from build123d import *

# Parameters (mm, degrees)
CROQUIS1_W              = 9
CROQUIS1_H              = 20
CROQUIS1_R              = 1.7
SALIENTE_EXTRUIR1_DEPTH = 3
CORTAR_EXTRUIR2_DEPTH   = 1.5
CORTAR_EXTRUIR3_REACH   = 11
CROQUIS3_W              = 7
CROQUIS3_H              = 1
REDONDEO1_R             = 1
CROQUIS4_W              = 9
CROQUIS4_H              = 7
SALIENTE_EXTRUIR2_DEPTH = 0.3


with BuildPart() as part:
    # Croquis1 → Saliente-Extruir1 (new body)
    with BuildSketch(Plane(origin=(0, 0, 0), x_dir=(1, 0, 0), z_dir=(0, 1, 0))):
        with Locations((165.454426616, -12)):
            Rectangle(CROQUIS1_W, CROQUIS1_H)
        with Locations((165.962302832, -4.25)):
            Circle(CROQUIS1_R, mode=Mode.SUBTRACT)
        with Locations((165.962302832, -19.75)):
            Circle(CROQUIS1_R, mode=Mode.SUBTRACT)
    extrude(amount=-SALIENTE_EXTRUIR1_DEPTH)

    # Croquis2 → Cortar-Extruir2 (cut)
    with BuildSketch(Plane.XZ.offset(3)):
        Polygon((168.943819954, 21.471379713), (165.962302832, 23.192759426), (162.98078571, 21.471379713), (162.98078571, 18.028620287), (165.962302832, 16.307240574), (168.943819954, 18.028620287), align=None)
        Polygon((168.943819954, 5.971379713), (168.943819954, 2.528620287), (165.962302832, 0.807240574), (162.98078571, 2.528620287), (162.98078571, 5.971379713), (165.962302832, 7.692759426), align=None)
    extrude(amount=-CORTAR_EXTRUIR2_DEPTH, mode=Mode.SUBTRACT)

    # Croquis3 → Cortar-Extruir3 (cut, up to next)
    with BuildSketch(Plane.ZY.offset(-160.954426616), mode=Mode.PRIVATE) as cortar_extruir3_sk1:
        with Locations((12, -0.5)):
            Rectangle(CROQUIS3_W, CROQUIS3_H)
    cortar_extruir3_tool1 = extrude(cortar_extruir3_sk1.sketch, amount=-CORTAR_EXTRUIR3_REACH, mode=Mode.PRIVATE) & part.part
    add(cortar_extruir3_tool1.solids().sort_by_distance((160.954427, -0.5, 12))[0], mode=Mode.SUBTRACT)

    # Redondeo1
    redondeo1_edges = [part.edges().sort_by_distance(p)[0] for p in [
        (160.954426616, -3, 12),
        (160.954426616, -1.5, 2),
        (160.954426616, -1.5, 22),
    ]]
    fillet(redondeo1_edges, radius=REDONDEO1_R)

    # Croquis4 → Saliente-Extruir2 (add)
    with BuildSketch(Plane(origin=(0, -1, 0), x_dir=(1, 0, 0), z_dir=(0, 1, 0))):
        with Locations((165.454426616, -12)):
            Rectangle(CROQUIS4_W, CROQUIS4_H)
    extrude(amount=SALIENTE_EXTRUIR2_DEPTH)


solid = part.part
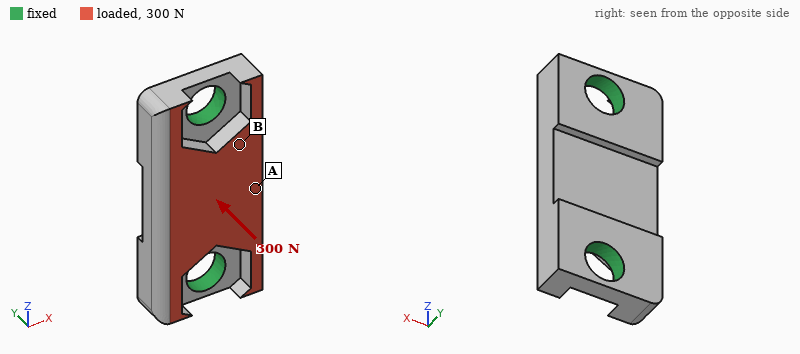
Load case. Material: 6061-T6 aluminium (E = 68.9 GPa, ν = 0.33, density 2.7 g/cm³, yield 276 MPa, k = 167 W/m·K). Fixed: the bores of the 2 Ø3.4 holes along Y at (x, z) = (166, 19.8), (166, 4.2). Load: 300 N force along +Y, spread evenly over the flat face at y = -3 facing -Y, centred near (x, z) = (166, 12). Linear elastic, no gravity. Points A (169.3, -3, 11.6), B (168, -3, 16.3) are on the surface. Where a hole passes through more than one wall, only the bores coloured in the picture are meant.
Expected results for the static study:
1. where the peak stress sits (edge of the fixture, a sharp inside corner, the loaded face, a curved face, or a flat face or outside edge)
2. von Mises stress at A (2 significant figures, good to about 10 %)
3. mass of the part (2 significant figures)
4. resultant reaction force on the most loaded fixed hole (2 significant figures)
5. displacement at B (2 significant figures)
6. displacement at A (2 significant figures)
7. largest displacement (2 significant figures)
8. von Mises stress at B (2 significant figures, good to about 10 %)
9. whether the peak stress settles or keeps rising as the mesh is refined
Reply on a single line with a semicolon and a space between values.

edge of the fixture; 28 MPa; 1.0 g; 190 N; 3.1 µm; 5.4 µm; 5.7 µm; 11 MPa; keeps rising
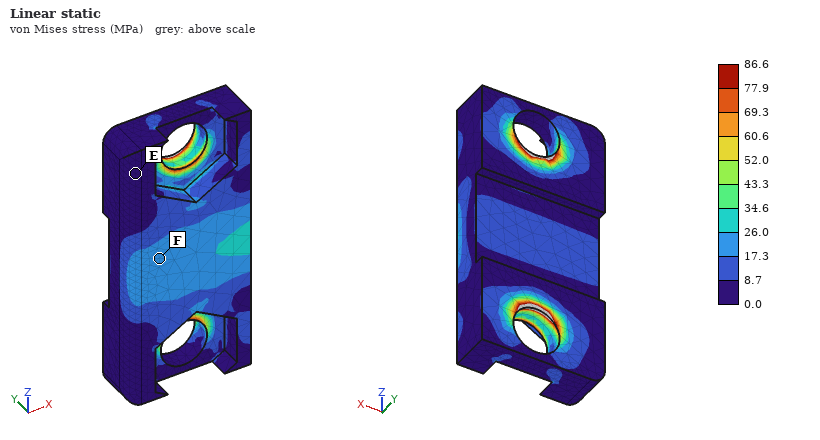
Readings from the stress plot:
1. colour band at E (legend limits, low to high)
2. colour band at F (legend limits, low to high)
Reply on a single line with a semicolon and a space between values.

0.0 to 8.7 MPa; 17.3 to 26.0 MPa
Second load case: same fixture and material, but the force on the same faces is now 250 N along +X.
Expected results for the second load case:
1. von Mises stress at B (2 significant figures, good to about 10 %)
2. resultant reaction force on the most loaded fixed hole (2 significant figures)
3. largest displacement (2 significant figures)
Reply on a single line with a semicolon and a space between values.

18 MPa; 130 N; 8.4 µm
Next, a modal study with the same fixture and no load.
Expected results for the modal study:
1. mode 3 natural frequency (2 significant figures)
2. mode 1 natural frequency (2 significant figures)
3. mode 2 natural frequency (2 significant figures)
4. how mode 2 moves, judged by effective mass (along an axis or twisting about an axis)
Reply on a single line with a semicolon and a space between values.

70 kHz; 38 kHz; 50 kHz; along Y
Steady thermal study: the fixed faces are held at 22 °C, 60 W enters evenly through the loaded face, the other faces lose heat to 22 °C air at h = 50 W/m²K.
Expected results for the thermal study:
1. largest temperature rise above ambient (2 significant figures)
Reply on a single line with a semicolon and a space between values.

46 K
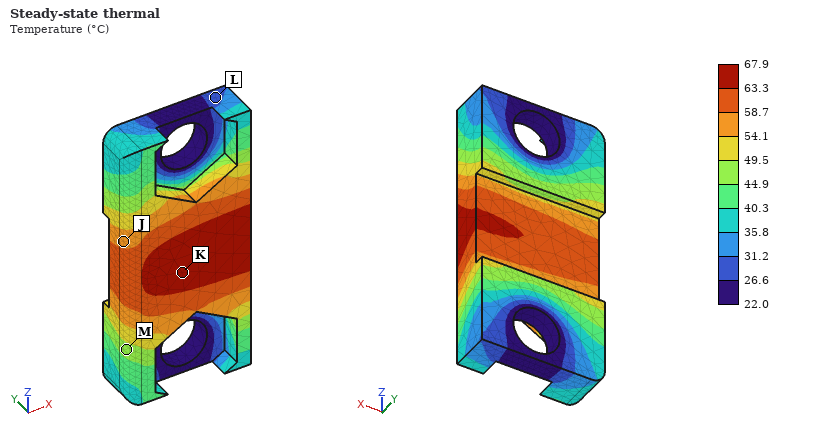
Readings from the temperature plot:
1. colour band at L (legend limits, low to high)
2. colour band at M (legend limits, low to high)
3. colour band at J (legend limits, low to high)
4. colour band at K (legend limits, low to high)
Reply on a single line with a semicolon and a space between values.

26.6 to 31.2 °C; 44.9 to 49.5 °C; 54.1 to 58.7 °C; 63.3 to 67.9 °C
